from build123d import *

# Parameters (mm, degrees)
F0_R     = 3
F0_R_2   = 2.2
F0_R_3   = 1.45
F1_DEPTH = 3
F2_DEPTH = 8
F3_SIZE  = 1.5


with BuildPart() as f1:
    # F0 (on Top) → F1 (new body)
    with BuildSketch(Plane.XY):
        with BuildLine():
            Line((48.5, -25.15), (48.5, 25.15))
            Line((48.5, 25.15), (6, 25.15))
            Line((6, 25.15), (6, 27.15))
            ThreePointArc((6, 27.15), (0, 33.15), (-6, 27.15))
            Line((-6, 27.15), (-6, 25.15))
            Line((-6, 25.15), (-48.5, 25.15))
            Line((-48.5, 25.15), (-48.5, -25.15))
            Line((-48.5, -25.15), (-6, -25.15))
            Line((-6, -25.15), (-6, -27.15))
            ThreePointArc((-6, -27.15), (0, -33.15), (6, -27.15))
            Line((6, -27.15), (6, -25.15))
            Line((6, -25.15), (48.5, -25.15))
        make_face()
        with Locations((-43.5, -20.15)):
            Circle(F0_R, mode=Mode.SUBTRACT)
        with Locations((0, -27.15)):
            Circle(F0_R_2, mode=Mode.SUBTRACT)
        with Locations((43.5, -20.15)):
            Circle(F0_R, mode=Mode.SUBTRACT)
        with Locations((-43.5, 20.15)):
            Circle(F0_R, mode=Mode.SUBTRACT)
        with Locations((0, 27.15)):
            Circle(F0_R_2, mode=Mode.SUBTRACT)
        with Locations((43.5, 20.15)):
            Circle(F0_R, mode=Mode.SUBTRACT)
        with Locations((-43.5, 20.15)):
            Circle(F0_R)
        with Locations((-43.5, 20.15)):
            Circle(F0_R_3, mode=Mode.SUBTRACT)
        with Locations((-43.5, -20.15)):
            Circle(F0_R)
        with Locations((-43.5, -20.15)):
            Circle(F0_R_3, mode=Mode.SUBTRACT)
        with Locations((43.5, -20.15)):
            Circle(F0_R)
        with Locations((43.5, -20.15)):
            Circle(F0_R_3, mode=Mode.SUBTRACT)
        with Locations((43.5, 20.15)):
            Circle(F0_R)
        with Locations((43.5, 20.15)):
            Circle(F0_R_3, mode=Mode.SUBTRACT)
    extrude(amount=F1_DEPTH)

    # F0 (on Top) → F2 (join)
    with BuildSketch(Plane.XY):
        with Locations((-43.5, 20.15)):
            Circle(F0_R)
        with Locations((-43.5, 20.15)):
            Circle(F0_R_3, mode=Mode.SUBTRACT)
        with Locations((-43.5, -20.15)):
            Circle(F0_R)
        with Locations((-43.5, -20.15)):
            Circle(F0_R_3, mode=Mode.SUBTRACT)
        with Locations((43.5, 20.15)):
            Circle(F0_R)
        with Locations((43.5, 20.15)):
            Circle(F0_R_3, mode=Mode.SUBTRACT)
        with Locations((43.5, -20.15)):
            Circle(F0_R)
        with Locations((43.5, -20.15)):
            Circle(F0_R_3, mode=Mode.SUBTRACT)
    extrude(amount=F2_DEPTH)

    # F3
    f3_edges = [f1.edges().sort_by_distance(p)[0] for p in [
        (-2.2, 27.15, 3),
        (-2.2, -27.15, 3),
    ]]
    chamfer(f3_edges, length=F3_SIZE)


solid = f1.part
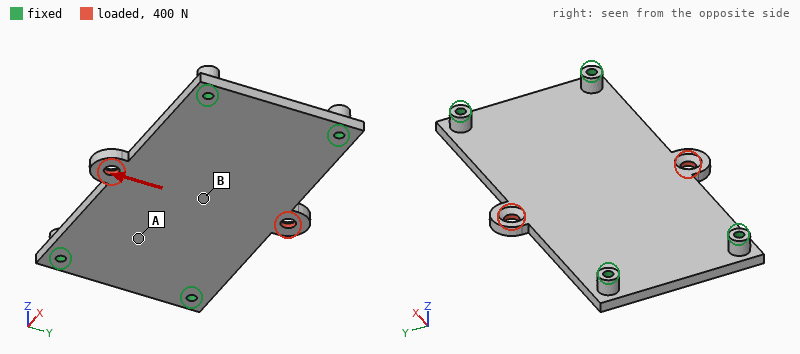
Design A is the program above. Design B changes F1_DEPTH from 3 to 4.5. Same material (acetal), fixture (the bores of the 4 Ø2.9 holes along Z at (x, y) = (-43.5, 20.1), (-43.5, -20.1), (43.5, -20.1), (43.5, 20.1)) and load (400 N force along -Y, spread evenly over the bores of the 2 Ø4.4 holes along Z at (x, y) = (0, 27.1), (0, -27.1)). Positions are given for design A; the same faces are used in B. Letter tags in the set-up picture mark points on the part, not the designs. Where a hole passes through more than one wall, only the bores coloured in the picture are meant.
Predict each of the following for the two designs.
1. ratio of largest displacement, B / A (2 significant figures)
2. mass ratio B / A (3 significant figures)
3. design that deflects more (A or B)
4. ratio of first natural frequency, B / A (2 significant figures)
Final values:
0.36
1.48
A
1.4
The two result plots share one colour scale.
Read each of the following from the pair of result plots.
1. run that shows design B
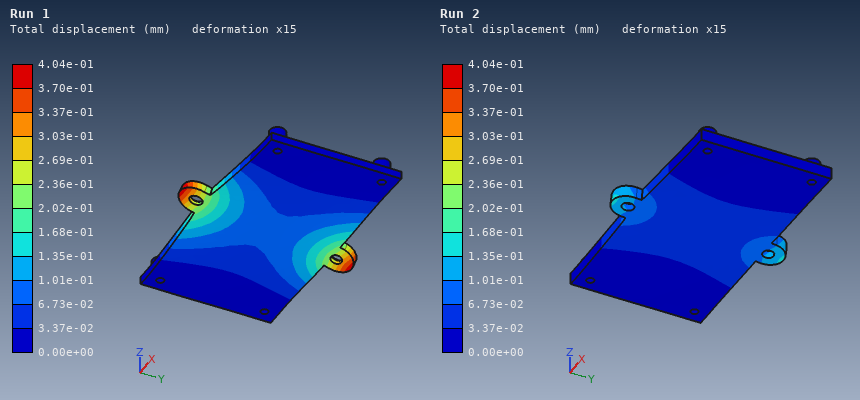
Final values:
Run 2
